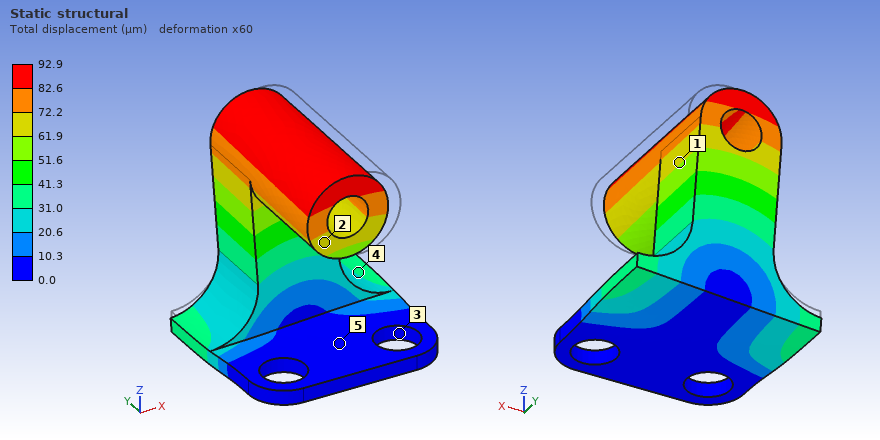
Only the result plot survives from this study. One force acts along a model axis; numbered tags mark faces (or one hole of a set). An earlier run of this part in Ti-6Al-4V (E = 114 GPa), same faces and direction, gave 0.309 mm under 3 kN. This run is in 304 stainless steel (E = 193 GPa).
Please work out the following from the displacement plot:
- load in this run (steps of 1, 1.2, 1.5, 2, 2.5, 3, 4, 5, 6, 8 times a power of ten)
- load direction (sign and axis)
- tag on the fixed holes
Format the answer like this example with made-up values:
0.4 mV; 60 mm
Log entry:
1.5 kN; -X; 3
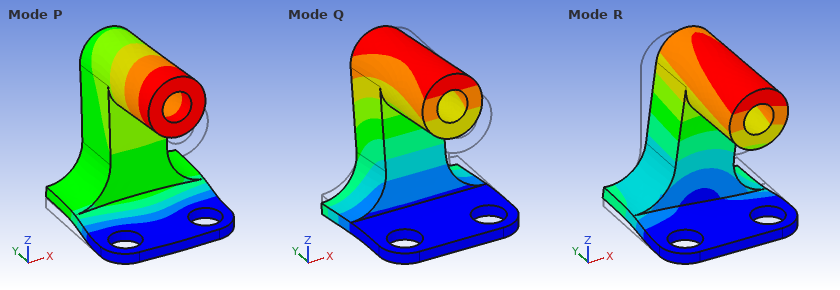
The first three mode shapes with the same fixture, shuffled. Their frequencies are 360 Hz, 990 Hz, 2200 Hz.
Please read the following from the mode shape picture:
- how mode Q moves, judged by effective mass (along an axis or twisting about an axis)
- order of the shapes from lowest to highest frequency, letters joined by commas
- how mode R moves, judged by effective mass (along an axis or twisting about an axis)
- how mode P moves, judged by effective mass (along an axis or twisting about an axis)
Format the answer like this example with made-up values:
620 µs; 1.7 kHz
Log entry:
along Y; Q, R, P; along X; along Z
